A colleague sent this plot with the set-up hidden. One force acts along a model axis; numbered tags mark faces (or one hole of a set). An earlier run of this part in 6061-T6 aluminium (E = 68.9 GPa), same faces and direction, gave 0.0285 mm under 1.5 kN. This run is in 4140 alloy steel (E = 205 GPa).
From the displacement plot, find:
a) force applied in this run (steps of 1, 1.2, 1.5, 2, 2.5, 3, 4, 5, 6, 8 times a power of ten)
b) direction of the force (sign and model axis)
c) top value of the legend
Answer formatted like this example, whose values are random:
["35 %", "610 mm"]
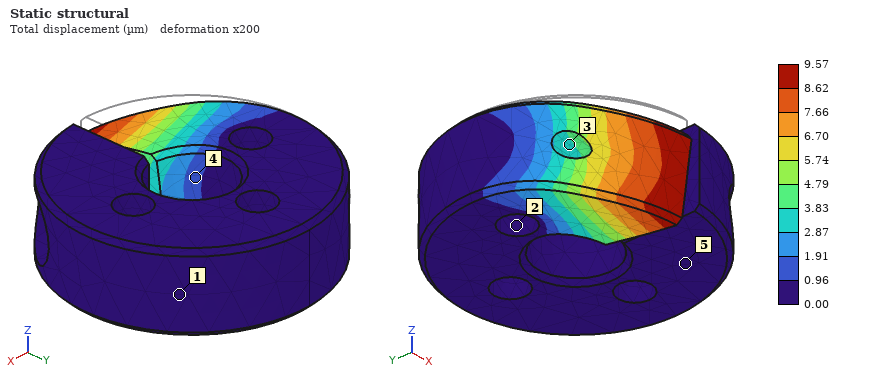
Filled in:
["1.5 kN", "-Z", "9.57 µm"]
